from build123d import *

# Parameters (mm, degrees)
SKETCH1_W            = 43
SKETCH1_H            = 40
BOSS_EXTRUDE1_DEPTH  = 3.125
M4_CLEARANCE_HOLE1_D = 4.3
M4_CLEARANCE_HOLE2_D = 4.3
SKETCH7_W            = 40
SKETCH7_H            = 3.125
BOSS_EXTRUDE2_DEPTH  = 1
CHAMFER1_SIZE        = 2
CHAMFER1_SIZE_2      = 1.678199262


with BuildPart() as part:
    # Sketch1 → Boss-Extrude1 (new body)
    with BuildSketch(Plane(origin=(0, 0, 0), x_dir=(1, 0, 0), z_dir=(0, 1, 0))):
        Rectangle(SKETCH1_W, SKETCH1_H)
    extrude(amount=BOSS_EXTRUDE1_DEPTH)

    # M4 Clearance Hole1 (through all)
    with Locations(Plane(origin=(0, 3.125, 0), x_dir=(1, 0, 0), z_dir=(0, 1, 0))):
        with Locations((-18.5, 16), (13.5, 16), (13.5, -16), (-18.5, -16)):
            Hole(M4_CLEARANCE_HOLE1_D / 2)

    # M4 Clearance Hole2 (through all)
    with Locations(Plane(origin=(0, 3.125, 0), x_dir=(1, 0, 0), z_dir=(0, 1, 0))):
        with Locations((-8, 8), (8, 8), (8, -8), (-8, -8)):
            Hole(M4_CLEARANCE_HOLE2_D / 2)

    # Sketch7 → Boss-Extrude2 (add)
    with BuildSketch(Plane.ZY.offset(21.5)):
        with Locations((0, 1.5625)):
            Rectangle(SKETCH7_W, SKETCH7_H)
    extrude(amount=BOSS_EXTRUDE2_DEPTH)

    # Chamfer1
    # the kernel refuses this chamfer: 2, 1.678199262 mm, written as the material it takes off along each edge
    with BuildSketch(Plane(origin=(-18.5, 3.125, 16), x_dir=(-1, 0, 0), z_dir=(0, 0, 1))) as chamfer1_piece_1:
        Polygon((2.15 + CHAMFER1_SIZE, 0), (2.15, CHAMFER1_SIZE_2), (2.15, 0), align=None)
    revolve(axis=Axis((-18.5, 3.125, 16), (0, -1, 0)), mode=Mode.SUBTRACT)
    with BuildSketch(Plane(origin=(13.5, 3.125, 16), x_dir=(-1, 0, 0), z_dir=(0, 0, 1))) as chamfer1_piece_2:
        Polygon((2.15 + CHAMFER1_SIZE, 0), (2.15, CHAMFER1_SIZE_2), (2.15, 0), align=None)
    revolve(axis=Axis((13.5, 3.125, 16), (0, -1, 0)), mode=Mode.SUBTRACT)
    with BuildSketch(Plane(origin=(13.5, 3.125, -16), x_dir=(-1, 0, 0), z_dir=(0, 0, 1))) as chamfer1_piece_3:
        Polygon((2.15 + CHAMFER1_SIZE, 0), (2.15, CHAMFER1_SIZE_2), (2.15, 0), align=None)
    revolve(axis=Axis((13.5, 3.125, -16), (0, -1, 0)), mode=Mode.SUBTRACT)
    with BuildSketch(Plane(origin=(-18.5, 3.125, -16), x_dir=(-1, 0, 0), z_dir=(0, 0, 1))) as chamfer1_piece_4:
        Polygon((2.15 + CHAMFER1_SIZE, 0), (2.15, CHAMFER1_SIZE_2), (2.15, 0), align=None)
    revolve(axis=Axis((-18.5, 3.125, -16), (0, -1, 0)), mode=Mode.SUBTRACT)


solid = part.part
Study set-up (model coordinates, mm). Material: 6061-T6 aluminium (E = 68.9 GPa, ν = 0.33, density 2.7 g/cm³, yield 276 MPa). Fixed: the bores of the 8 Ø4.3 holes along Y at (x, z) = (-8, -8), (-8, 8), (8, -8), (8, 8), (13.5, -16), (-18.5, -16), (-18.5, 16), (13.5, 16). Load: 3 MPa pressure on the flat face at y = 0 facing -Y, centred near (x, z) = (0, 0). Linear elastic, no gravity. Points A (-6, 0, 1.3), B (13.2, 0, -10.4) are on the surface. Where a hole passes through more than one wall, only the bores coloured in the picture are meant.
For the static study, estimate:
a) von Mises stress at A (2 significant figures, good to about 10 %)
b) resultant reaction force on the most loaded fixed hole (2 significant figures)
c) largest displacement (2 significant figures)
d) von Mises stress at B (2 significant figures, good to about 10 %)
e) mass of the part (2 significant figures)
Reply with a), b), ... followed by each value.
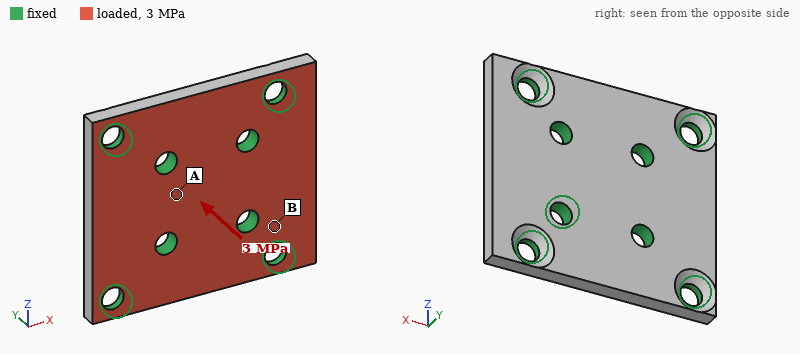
a) 20 MPa
b) 850 N
c) 41 µm
d) 53 MPa
e) 14 g
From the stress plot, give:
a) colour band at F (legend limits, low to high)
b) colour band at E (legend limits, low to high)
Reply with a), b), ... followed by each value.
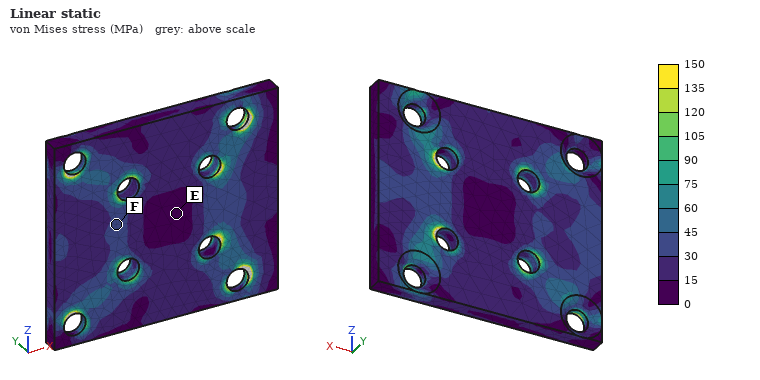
a) 30 to 45 MPa
b) 0 to 15 MPa
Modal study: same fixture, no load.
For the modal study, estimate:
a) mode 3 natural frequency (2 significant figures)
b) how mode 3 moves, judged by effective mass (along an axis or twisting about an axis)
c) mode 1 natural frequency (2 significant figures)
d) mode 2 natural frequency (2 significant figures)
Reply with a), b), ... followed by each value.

a) 26 kHz
b) twisting about X
c) 20 kHz
d) 22 kHz
